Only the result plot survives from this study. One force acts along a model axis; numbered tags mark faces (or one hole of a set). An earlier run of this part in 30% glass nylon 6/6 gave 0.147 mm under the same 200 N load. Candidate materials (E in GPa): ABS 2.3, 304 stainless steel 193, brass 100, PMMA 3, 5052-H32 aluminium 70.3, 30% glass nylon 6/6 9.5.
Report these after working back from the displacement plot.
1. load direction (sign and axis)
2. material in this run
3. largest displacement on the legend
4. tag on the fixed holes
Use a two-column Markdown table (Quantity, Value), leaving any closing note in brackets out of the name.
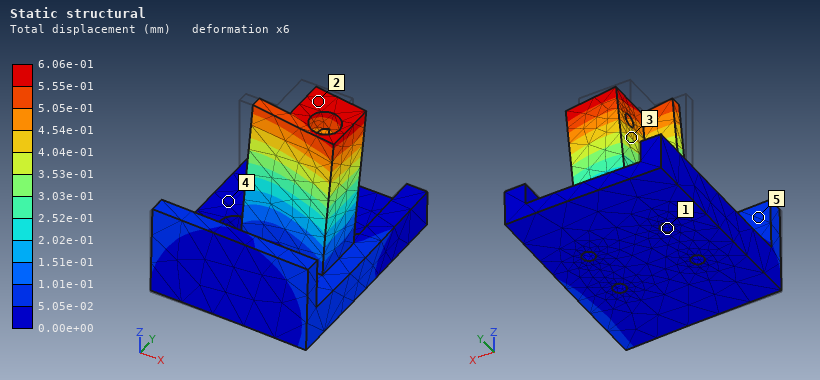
| Quantity | Value |
|---|---|
| load direction | +X |
| material in this run | ABS |
| largest displacement on the legend | 6.06e-01 mm |
| tag on the fixed holes | 1 |
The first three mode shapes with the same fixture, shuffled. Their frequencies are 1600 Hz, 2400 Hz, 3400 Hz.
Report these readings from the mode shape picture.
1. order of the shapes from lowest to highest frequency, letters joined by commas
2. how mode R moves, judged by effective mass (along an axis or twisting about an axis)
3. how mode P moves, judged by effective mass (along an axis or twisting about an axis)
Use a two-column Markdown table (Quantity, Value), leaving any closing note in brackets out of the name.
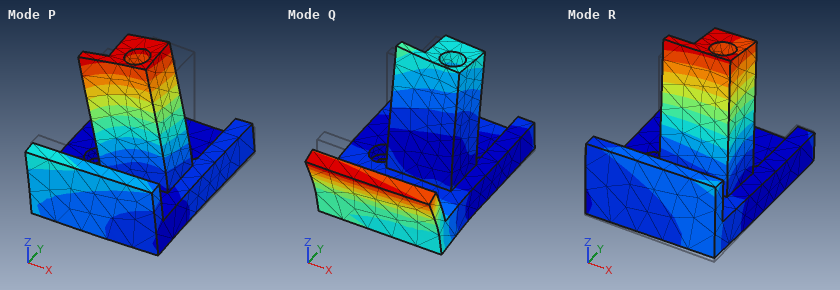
| Quantity | Value |
|---|---|
| order of the shapes from lowest to highest frequency, letters joined by commas | R, P, Q |
| how mode R moves, judged by effective mass | along Y |
| how mode P moves, judged by effective mass | along X |
